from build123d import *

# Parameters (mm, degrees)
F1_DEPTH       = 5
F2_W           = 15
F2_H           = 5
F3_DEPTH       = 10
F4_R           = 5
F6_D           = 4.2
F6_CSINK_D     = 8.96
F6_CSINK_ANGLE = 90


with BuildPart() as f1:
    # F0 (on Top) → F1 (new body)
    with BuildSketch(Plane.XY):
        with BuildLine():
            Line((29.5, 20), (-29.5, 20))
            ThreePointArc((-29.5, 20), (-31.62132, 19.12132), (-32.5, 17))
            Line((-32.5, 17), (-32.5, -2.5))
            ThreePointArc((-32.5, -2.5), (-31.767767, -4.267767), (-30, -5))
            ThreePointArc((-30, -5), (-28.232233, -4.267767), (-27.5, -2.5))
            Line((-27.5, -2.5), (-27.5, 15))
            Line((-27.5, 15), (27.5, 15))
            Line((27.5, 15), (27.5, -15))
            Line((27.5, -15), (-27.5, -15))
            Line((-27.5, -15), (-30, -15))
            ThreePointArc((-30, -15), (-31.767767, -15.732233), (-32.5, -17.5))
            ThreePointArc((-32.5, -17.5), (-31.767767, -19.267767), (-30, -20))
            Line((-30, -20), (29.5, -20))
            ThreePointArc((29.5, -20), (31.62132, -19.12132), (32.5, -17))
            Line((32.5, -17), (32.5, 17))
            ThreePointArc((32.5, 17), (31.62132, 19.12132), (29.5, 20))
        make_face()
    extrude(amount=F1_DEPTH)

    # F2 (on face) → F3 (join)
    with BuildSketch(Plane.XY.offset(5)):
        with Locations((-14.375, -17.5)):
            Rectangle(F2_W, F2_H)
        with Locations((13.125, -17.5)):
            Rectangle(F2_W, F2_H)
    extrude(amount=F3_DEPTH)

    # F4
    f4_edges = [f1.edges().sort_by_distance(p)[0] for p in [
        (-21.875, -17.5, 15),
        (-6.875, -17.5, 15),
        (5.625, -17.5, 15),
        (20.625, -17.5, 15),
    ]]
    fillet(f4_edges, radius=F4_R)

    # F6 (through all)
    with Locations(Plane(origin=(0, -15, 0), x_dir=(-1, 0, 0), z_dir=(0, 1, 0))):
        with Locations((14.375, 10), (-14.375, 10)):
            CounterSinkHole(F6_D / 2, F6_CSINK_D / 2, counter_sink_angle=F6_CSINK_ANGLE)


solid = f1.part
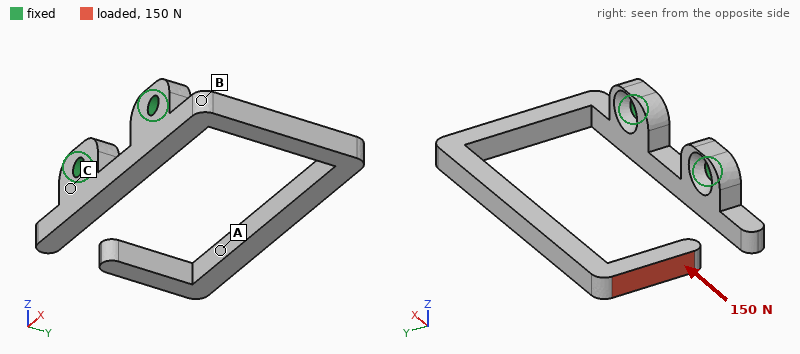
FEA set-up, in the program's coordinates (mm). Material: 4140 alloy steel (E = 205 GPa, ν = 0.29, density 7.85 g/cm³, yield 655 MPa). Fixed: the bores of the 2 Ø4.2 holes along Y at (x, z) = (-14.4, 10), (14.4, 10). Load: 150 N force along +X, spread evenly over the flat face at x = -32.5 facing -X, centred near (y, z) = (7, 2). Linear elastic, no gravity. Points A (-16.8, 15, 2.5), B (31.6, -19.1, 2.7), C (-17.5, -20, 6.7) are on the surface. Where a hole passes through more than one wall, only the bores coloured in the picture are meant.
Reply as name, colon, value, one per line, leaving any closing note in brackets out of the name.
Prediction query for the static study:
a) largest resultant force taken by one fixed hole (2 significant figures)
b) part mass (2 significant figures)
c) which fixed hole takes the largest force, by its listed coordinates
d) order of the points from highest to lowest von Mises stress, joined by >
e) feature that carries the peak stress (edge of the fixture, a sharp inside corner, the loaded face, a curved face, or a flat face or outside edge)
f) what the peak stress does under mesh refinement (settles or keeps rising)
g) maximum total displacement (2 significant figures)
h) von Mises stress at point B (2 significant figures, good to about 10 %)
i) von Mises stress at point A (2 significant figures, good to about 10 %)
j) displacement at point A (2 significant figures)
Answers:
largest resultant force taken by one fixed hole: 110 N
part mass: 44 g
which fixed hole takes the largest force, by its listed coordinates: (-14.4, 10)
order of the points from highest to lowest von Mises stress, joined by >: A > B > C
feature that carries the peak stress: edge of the fixture
what the peak stress does under mesh refinement: keeps rising
maximum total displacement: 0.37 mm
von Mises stress at point B: 34 MPa
von Mises stress at point A: 80 MPa
displacement at point A: 0.35 mm
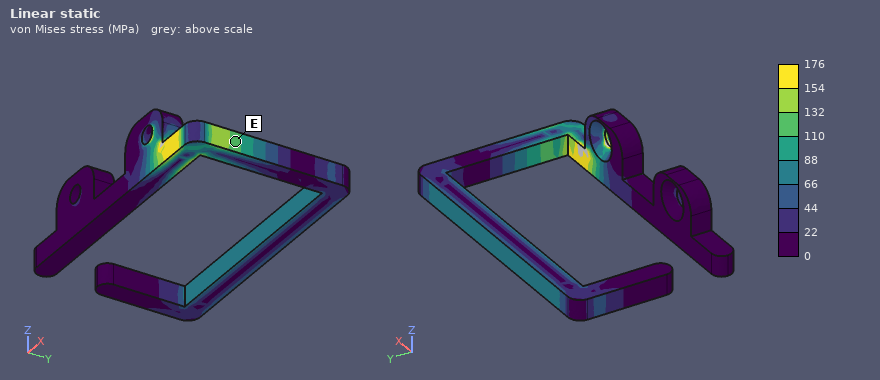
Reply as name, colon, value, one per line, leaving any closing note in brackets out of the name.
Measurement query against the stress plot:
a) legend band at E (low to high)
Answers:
legend band at E: 110 to 132 MPa
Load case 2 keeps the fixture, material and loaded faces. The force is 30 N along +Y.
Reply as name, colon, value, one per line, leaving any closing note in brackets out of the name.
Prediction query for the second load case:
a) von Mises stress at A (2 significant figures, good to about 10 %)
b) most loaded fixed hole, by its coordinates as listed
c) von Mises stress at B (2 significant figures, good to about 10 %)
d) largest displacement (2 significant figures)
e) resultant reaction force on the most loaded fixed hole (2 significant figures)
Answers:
von Mises stress at A: 23 MPa
most loaded fixed hole, by its coordinates as listed: (-14.4, 10)
von Mises stress at B: 18 MPa
largest displacement: 0.73 mm
resultant reaction force on the most loaded fixed hole: 26 N
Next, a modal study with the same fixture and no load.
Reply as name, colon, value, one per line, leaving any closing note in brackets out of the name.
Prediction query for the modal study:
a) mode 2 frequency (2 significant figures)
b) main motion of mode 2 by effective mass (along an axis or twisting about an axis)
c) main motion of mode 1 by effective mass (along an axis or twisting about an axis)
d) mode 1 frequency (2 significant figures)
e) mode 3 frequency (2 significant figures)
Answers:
mode 2 frequency: 360 Hz
main motion of mode 2 by effective mass: along Y
main motion of mode 1 by effective mass: along Z
mode 1 frequency: 330 Hz
mode 3 frequency: 1000 Hz
